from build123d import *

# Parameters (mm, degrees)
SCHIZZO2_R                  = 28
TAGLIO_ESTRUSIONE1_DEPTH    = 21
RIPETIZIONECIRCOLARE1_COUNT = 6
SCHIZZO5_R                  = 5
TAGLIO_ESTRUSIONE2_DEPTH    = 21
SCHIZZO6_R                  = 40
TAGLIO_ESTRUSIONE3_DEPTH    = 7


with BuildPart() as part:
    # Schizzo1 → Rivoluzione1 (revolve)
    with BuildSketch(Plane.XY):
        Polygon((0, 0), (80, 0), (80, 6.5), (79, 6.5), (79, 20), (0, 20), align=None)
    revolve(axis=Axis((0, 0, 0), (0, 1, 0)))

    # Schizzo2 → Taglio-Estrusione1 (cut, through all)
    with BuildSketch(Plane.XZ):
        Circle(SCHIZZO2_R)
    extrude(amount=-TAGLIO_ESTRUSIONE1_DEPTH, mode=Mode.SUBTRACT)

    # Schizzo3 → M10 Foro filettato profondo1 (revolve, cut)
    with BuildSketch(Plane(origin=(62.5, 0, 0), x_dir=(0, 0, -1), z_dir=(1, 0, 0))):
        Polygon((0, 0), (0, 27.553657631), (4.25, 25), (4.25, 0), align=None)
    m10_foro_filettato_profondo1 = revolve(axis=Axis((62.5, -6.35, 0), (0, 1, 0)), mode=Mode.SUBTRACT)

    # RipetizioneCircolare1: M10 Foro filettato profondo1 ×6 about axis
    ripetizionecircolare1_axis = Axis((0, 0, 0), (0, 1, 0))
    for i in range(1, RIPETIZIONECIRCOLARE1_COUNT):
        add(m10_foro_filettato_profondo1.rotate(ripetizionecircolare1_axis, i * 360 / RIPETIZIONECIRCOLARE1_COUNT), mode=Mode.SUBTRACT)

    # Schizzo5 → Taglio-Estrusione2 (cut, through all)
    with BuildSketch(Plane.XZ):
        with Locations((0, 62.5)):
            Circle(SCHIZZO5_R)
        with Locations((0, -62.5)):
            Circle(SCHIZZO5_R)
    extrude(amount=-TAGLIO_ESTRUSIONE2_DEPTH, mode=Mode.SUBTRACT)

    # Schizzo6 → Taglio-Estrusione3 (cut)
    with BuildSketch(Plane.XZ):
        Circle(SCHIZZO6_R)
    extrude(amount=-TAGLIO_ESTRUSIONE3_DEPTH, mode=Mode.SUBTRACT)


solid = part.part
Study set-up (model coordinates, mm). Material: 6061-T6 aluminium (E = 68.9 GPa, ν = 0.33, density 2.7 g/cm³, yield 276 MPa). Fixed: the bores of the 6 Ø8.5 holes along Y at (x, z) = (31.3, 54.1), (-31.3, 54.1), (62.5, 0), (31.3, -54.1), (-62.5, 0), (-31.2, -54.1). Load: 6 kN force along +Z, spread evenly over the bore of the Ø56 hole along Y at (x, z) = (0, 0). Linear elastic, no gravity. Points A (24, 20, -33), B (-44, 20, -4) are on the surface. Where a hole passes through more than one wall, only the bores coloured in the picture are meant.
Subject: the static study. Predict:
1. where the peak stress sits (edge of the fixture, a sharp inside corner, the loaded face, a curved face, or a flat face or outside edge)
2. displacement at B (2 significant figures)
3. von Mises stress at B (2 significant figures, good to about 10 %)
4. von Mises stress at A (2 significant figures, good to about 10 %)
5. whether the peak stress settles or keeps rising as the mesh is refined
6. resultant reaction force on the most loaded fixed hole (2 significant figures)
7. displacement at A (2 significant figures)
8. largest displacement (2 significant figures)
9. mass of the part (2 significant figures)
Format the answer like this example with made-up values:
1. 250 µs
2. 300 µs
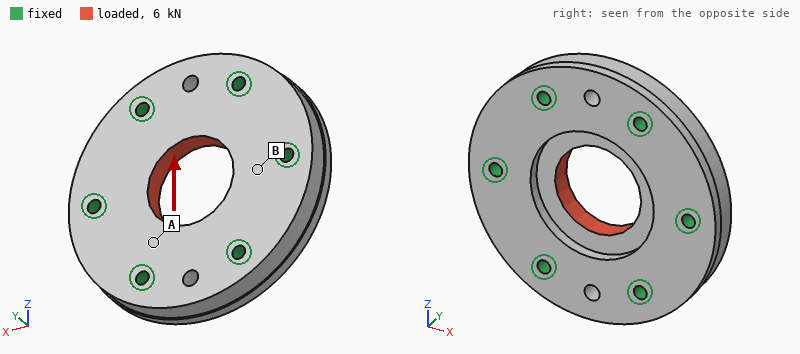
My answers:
1. edge of the fixture
2. 0.54 µm
3. 0.60 MPa
4. 2.8 MPa
5. keeps rising
6. 1.3 kN
7. 1.0 µm
8. 2.0 µm
9. 860 g
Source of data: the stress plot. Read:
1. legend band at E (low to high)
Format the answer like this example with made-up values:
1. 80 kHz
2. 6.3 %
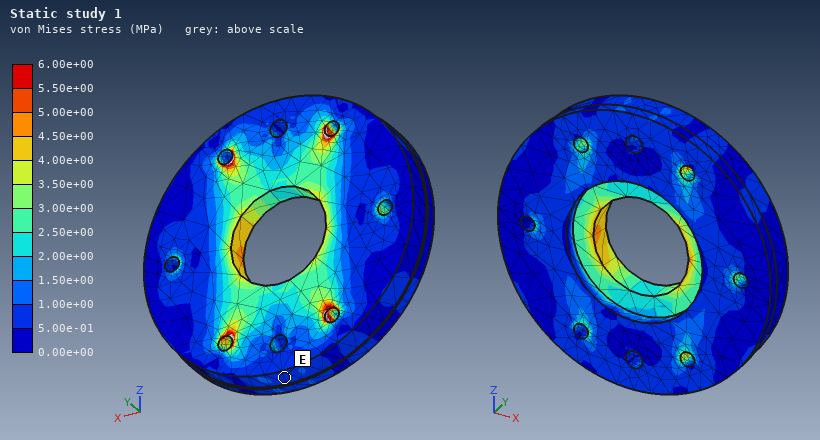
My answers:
1. 5.00e-01 to 1.00e+00 MPa
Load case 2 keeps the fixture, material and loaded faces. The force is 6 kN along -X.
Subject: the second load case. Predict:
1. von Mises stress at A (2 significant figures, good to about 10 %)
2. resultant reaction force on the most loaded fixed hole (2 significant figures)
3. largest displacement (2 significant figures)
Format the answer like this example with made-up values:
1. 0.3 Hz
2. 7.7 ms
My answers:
1. 1.7 MPa
2. 1.4 kN
3. 1.9 µm
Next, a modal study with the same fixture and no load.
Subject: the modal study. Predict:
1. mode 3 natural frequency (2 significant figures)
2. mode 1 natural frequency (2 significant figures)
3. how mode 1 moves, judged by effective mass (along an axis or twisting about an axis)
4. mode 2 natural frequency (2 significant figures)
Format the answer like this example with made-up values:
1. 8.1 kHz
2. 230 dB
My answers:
1. 14 kHz
2. 12 kHz
3. along Y
4. 14 kHz
